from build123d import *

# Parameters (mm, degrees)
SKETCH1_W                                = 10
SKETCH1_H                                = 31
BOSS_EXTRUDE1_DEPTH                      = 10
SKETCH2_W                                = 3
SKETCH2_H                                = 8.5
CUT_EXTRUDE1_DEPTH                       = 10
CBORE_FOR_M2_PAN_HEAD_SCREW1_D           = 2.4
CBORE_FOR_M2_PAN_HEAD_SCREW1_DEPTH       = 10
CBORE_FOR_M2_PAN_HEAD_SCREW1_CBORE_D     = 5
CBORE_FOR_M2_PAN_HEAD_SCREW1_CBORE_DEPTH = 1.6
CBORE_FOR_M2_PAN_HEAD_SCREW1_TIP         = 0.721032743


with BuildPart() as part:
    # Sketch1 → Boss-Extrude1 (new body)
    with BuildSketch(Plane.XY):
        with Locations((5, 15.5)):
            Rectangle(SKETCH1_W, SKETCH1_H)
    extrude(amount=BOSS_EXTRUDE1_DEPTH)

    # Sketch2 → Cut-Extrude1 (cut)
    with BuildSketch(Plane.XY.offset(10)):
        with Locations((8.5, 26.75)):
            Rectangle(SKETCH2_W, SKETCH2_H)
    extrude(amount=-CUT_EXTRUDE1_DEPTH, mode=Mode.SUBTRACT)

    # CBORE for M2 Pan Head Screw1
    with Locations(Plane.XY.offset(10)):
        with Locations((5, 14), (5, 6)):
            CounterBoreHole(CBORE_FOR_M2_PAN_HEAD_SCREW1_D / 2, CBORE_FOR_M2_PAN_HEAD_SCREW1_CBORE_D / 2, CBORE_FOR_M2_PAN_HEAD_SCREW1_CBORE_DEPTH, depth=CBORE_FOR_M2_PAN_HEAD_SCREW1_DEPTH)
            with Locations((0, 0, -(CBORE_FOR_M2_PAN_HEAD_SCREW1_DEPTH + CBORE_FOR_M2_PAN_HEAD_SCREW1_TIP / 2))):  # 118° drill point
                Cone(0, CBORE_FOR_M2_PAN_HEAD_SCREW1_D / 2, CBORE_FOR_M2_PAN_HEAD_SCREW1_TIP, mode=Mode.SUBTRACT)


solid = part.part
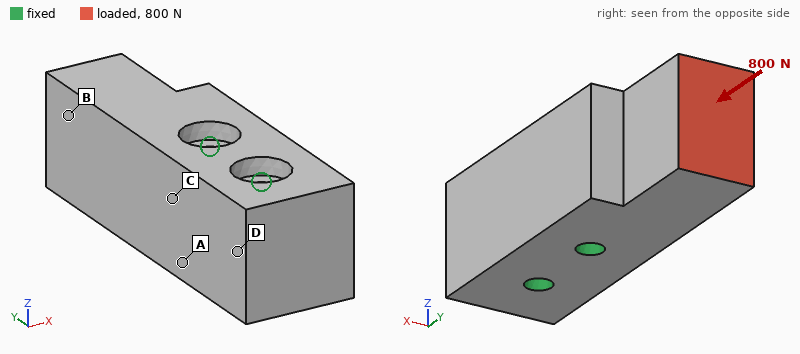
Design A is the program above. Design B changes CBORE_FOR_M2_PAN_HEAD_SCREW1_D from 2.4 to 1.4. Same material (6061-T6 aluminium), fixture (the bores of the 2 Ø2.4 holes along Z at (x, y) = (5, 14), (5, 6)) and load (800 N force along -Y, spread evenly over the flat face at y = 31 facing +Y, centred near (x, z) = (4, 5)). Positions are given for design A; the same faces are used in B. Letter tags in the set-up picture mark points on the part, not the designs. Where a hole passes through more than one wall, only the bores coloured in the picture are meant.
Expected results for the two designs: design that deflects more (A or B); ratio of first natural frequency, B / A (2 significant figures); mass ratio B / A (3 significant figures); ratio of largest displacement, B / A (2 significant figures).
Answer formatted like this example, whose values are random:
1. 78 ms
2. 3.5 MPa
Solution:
1. B
2. 0.91
3. 1.02
4. 1.1
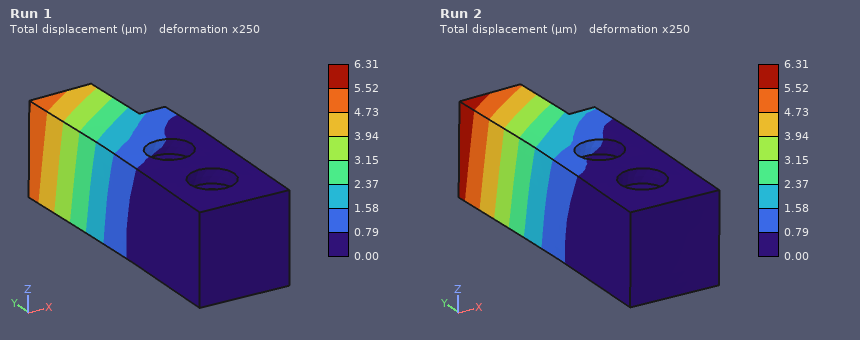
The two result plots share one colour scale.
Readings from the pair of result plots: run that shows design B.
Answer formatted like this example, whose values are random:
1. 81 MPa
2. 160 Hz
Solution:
1. Run 2
